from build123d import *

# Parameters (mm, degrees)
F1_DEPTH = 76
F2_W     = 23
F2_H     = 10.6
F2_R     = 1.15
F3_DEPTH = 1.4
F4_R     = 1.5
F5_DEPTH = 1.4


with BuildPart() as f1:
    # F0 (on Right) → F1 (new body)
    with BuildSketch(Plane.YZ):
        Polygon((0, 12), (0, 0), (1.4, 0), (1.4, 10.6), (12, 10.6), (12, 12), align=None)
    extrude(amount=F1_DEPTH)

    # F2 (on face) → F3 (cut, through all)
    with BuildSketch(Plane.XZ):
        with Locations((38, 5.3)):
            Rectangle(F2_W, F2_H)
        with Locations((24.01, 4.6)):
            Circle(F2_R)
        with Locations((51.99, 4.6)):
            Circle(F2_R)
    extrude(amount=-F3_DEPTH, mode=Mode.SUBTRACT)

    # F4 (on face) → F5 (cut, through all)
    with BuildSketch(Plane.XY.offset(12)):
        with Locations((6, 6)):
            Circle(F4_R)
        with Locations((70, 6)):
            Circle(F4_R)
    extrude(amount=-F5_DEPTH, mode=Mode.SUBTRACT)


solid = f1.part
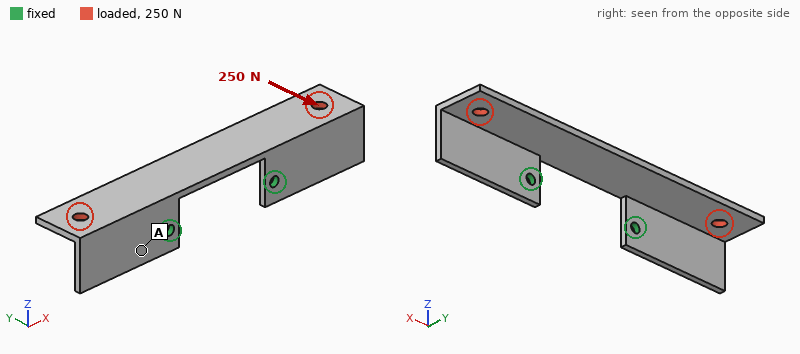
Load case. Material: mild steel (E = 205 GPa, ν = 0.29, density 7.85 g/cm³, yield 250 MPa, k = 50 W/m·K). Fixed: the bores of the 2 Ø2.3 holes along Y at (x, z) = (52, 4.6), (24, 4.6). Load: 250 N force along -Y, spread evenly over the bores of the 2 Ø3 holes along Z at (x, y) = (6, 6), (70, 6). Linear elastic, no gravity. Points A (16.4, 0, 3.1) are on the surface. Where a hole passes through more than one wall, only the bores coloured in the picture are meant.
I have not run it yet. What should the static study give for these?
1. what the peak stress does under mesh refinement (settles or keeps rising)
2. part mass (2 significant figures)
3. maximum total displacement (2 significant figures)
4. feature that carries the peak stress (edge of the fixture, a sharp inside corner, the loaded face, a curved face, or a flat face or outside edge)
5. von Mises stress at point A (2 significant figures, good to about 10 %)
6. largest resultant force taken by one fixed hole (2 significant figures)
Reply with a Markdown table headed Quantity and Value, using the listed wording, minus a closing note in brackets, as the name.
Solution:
| Quantity | Value |
|---|---|
| what the peak stress does under mesh refinement | keeps rising |
| part mass | 16 g |
| maximum total displacement | 76 µm |
| feature that carries the peak stress | edge of the fixture |
| von Mises stress at point A | 42 MPa |
| largest resultant force taken by one fixed hole | 150 N |
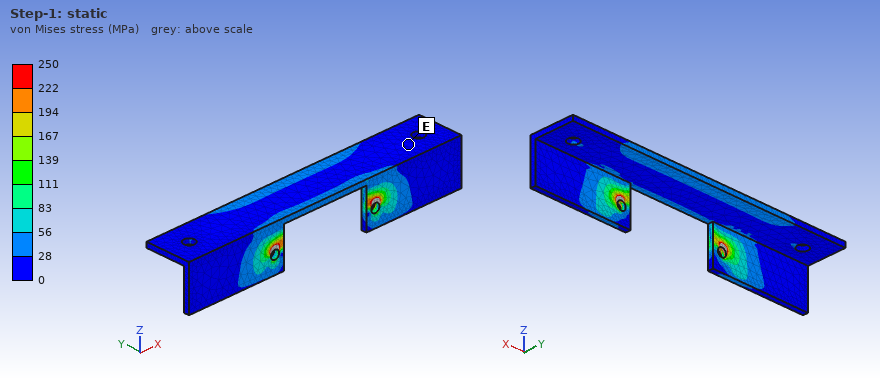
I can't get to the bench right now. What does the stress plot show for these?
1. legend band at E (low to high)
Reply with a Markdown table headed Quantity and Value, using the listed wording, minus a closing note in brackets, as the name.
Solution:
| Quantity | Value |
|---|---|
| legend band at E | 0 to 28 MPa |
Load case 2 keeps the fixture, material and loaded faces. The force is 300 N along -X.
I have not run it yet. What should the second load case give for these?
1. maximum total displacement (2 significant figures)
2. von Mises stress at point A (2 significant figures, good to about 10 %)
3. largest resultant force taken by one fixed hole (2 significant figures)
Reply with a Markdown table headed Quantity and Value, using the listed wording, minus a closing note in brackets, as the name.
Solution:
| Quantity | Value |
|---|---|
| maximum total displacement | 27 µm |
| von Mises stress at point A | 19 MPa |
| largest resultant force taken by one fixed hole | 160 N |
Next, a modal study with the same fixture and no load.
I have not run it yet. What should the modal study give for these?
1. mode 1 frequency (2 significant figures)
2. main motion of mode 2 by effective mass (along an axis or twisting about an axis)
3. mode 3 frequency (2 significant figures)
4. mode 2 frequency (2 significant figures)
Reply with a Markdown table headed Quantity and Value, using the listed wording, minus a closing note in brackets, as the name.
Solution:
| Quantity | Value |
|---|---|
| mode 1 frequency | 2800 Hz |
| main motion of mode 2 by effective mass | twisting about Z |
| mode 3 frequency | 4200 Hz |
| mode 2 frequency | 3000 Hz |
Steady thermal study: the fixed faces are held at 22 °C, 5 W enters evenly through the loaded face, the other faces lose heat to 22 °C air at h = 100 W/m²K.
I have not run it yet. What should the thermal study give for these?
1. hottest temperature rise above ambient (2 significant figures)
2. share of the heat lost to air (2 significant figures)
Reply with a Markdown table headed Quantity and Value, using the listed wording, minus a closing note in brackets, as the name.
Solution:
| Quantity | Value |
|---|---|
| hottest temperature rise above ambient | 29 K |
| share of the heat lost to air | 67 % |
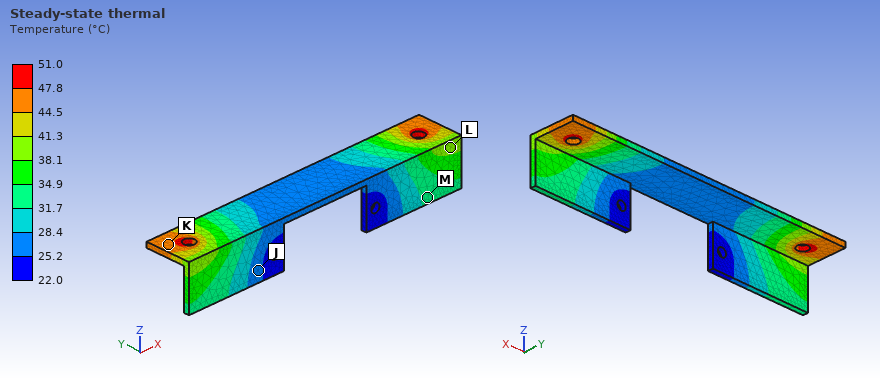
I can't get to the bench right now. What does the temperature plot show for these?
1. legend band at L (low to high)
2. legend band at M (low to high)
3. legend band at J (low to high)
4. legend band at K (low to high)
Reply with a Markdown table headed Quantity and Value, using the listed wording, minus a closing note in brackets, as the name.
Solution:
| Quantity | Value |
|---|---|
| legend band at L | 38.1 to 41.3 °C |
| legend band at M | 31.7 to 34.9 °C |
| legend band at J | 25.2 to 28.4 °C |
| legend band at K | 44.5 to 47.8 °C |
